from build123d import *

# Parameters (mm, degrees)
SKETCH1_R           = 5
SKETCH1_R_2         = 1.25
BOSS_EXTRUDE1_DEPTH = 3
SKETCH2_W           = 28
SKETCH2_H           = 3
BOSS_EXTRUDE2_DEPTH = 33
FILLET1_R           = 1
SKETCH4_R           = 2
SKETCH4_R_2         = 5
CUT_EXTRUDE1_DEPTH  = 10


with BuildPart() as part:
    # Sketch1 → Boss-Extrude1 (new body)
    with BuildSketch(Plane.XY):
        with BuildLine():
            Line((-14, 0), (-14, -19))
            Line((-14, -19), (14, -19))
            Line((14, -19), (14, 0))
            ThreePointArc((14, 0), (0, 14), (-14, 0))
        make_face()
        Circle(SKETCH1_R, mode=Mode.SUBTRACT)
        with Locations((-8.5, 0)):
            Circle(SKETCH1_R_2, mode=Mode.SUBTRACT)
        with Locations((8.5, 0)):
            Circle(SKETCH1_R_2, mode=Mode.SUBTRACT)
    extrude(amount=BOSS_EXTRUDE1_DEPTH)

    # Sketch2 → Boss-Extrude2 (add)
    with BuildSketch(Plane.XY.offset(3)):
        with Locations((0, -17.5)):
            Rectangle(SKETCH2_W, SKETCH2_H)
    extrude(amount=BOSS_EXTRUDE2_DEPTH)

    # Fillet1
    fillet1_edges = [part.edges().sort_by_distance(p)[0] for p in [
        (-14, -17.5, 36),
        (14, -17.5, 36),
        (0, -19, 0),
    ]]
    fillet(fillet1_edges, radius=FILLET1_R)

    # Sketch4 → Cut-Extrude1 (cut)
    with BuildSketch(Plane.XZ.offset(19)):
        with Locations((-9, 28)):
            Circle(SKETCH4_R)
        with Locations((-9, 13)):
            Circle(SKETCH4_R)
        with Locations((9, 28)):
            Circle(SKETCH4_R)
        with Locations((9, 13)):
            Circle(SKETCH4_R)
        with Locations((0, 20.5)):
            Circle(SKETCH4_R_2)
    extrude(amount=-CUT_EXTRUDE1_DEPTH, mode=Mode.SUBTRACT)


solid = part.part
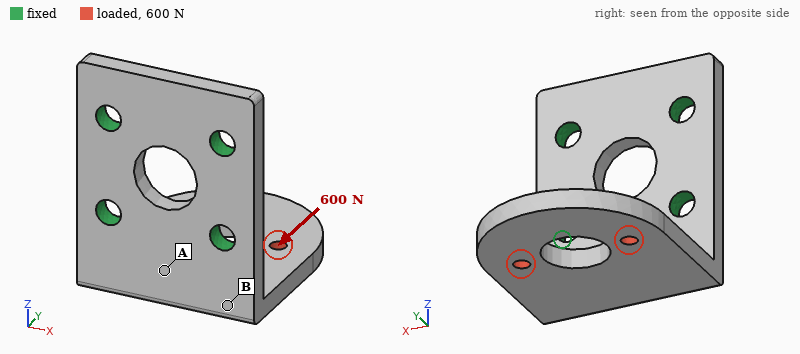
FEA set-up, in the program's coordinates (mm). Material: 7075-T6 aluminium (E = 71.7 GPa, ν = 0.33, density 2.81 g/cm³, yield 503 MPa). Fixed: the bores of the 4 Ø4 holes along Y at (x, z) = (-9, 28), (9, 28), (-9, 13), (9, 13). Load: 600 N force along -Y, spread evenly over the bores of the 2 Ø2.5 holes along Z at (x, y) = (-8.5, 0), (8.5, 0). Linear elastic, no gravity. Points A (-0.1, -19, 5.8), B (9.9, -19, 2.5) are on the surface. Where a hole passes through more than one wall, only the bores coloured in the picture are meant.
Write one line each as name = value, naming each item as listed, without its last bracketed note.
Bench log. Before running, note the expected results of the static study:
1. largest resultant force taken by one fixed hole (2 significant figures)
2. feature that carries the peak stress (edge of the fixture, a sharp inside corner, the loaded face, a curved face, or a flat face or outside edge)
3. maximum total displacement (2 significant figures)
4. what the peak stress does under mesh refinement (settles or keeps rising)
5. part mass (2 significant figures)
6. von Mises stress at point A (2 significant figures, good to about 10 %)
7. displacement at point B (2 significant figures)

largest resultant force taken by one fixed hole = 320 N
feature that carries the peak stress = edge of the fixture
maximum total displacement = 0.25 mm
what the peak stress does under mesh refinement = keeps rising
part mass = 13 g
von Mises stress at point A = 49 MPa
displacement at point B = 0.051 mm
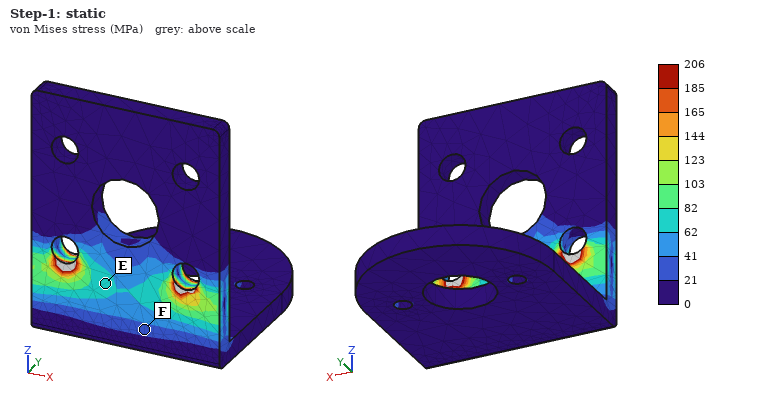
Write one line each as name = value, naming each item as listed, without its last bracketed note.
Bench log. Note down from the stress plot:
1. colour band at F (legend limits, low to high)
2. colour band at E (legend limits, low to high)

colour band at F = 21 to 41 MPa
colour band at E = 62 to 82 MPa
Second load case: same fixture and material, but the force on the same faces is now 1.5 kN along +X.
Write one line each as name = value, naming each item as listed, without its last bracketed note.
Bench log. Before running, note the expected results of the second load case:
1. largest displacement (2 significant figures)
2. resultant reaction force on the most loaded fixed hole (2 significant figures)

largest displacement = 0.45 mm
resultant reaction force on the most loaded fixed hole = 1.7 kN
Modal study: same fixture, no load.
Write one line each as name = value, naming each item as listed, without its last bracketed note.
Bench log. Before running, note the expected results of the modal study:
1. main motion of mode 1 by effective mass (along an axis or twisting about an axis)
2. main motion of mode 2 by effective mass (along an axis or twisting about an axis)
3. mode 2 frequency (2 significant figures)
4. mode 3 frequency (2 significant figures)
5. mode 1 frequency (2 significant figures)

main motion of mode 1 by effective mass = along Z
main motion of mode 2 by effective mass = along X
mode 2 frequency = 4600 Hz
mode 3 frequency = 7500 Hz
mode 1 frequency = 2000 Hz
